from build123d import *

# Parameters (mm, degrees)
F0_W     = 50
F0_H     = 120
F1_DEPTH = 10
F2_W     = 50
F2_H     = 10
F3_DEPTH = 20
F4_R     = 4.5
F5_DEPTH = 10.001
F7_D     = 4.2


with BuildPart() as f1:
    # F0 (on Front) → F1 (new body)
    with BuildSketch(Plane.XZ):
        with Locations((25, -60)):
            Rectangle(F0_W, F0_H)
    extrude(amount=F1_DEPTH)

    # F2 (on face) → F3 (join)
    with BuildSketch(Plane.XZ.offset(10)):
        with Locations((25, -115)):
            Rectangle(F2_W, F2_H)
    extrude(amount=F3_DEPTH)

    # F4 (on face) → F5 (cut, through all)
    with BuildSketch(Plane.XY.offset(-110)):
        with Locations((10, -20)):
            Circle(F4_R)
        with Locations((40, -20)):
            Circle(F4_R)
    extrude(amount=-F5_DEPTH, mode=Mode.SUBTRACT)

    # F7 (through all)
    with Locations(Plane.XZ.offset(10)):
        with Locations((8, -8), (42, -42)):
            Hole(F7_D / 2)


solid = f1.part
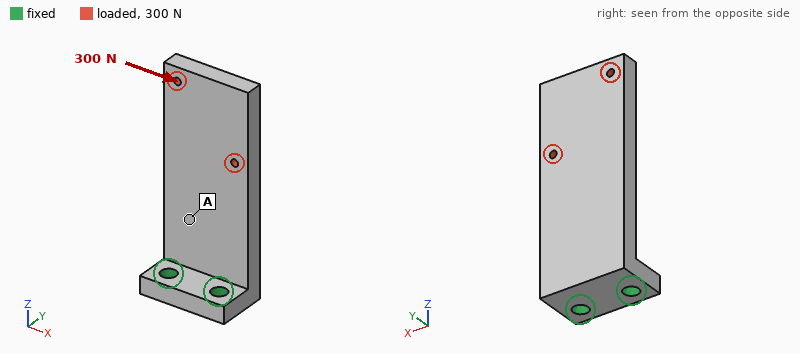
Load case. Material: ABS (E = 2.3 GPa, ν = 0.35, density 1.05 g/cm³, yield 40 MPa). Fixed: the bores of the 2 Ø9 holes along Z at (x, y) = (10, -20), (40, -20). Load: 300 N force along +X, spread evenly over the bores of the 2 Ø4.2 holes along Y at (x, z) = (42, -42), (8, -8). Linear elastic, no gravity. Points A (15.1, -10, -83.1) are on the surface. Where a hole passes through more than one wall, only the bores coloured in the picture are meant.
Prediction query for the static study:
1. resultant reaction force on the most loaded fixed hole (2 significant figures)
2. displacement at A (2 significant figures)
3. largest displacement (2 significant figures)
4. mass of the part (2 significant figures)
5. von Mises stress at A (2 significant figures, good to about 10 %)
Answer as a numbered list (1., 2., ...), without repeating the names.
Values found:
1. 770 N
2. 0.31 mm
3. 1.3 mm
4. 72 g
5. 2.9 MPa
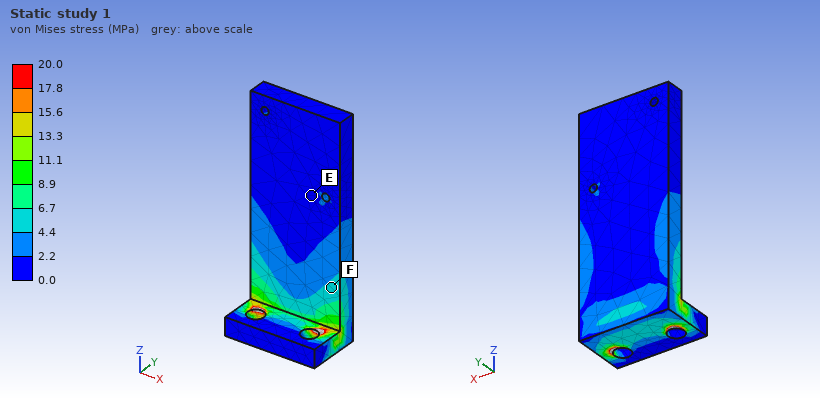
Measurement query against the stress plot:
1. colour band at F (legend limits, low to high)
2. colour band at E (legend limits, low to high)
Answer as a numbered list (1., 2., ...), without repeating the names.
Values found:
1. 4.4 to 6.7 MPa
2. 0.0 to 2.2 MPa
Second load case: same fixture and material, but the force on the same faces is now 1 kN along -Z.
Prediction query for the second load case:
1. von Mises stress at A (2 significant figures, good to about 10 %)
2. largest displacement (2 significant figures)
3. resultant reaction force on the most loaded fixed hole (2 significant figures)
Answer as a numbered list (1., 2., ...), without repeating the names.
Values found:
1. 2.0 MPa
2. 1.2 mm
3. 500 N
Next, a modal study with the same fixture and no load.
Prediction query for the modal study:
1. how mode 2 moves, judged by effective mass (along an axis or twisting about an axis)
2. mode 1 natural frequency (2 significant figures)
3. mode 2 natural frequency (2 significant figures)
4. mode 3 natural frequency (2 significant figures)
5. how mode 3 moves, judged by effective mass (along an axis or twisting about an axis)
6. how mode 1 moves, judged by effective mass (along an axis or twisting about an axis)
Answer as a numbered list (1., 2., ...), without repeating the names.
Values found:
1. along X
2. 160 Hz
3. 490 Hz
4. 800 Hz
5. twisting about Z
6. along Y
